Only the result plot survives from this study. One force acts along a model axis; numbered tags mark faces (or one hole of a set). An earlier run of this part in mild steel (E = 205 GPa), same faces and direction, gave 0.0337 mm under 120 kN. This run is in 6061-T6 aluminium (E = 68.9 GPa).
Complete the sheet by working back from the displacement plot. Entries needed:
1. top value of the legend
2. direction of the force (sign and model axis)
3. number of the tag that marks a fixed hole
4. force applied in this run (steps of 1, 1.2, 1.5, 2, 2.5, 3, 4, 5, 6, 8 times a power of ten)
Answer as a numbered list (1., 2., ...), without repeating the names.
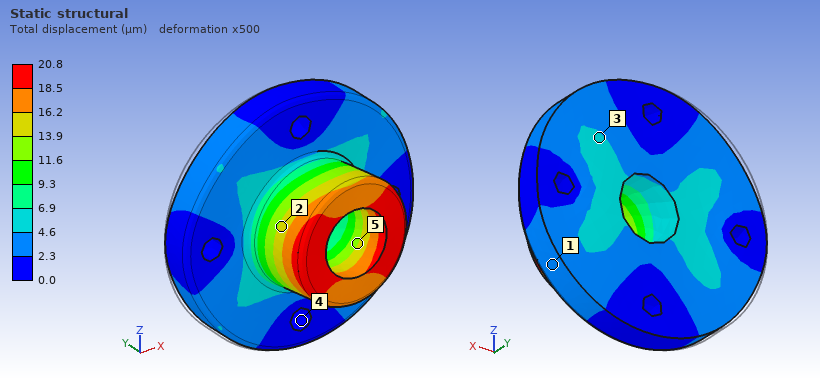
1. 20.8 µm
2. +X
3. 4
4. 25 kN
